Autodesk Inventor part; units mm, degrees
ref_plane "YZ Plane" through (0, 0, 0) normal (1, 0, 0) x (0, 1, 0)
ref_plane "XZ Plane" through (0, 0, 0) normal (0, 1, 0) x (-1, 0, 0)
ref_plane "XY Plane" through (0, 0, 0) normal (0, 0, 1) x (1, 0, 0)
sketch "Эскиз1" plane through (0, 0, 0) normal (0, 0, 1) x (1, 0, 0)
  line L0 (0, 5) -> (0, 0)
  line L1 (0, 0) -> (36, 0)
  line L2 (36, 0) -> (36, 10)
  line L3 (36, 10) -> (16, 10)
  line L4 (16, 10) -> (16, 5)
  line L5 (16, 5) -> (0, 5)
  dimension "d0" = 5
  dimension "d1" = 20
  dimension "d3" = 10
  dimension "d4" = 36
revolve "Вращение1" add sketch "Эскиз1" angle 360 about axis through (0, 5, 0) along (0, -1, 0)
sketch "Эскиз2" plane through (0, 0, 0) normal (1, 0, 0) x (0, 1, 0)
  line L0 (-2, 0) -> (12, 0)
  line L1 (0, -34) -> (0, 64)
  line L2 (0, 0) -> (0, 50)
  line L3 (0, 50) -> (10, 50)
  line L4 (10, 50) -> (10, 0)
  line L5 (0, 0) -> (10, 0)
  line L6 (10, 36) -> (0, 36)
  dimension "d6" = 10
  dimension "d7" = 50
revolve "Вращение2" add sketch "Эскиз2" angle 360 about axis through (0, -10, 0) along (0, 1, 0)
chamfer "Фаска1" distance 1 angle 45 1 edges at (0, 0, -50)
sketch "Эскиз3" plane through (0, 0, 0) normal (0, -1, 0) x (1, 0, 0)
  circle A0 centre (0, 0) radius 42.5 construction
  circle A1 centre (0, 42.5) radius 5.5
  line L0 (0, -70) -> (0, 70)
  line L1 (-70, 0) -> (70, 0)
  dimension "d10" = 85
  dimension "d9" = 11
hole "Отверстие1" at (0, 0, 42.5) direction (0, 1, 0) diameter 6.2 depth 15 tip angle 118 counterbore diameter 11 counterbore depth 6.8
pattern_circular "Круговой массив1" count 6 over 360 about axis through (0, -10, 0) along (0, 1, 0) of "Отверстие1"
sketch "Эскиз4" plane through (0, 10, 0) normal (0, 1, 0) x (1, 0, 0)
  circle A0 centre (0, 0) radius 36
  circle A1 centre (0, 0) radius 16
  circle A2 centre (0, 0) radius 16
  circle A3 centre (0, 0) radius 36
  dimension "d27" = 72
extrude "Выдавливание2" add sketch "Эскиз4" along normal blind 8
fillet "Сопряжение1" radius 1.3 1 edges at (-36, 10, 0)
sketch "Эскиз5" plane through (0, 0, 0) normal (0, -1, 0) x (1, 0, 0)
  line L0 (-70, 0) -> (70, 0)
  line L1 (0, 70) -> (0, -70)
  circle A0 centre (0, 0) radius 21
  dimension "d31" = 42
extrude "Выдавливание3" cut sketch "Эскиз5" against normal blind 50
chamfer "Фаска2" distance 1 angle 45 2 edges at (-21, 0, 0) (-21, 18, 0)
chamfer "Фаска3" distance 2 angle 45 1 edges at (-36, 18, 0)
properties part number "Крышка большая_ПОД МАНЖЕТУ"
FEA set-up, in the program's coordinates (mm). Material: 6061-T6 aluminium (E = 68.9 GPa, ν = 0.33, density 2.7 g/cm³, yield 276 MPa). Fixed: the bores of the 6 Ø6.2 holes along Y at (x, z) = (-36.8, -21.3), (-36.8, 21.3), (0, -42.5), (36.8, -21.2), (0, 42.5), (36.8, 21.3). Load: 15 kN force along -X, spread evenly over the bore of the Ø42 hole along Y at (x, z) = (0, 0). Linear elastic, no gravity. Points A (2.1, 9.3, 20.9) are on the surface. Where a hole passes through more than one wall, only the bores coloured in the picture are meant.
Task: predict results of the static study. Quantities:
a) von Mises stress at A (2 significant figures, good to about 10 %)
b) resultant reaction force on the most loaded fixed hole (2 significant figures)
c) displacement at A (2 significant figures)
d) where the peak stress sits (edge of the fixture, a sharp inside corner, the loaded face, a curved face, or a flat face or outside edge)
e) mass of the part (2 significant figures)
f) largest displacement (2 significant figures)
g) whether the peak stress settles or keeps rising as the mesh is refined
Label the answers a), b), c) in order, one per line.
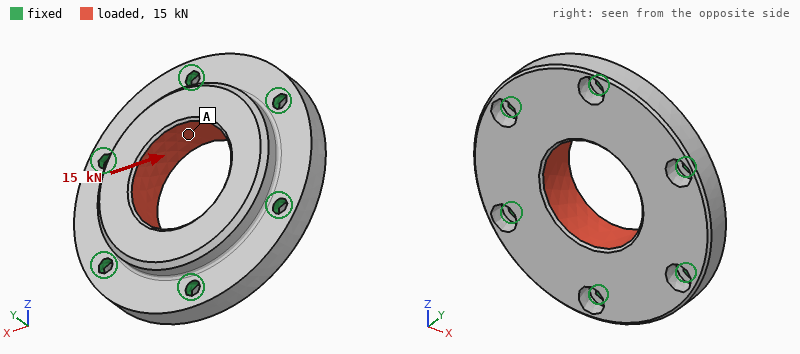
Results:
a) 12 MPa
b) 2.8 kN
c) 7.3 µm
d) edge of the fixture
e) 220 g
f) 8.2 µm
g) keeps rising
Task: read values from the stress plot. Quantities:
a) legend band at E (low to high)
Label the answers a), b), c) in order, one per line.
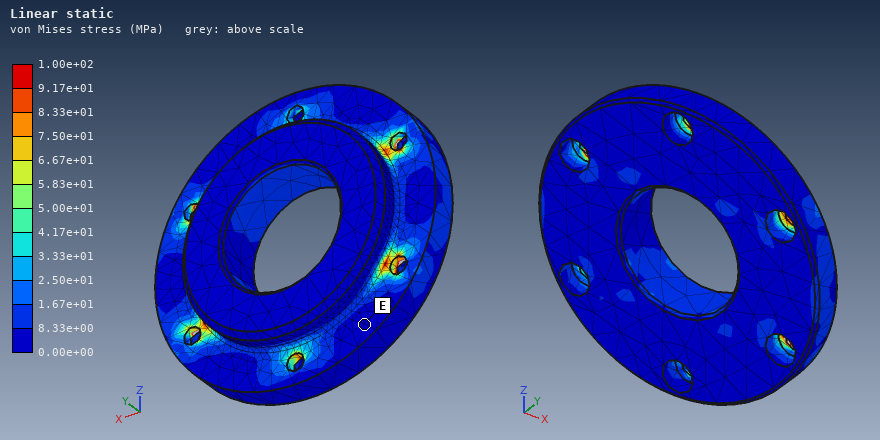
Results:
a) 0.00e+00 to 8.33e+00 MPa
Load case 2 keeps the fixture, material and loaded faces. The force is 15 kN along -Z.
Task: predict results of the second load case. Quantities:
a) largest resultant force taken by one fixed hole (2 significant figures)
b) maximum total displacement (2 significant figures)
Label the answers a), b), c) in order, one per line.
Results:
a) 3.1 kN
b) 7.9 µm
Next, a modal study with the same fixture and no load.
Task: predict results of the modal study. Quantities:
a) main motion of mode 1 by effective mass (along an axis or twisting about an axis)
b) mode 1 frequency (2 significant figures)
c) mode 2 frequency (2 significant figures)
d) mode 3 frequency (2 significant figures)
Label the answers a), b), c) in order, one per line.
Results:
a) along Y
b) 10 kHz
c) 14 kHz
d) 14 kHz
